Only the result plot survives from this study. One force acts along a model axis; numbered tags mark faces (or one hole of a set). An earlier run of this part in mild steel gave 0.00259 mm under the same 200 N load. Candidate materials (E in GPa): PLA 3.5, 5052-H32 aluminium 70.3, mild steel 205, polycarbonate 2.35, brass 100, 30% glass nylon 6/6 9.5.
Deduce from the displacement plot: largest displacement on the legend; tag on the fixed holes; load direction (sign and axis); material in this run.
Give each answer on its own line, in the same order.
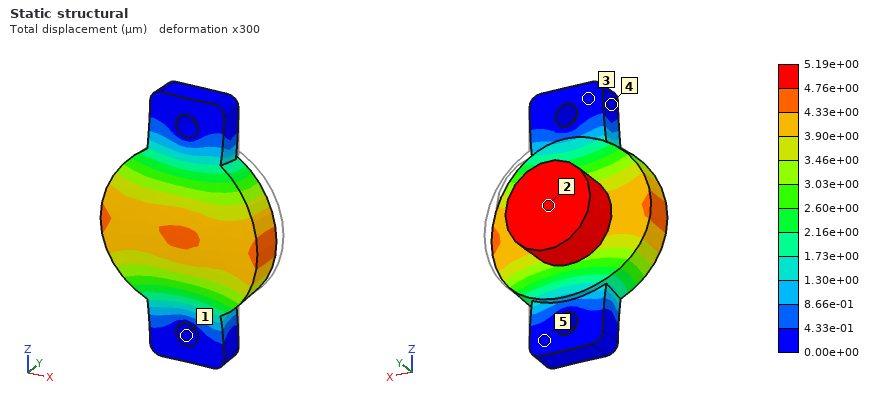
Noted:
5.19e+00 µm
1
-Y
brass
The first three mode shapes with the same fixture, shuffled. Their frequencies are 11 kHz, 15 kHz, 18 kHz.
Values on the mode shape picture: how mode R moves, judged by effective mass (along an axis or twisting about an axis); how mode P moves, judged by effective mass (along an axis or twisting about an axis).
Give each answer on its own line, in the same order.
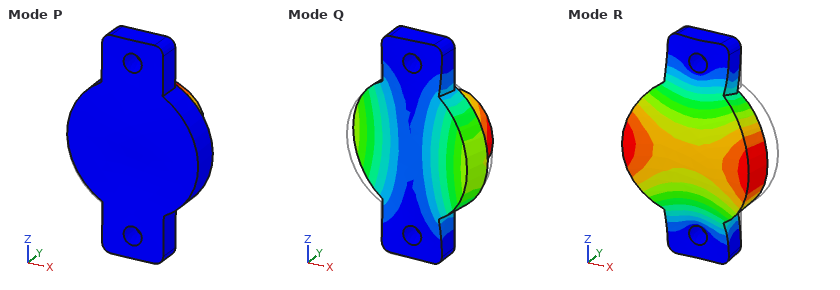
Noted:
along Y
along Z
